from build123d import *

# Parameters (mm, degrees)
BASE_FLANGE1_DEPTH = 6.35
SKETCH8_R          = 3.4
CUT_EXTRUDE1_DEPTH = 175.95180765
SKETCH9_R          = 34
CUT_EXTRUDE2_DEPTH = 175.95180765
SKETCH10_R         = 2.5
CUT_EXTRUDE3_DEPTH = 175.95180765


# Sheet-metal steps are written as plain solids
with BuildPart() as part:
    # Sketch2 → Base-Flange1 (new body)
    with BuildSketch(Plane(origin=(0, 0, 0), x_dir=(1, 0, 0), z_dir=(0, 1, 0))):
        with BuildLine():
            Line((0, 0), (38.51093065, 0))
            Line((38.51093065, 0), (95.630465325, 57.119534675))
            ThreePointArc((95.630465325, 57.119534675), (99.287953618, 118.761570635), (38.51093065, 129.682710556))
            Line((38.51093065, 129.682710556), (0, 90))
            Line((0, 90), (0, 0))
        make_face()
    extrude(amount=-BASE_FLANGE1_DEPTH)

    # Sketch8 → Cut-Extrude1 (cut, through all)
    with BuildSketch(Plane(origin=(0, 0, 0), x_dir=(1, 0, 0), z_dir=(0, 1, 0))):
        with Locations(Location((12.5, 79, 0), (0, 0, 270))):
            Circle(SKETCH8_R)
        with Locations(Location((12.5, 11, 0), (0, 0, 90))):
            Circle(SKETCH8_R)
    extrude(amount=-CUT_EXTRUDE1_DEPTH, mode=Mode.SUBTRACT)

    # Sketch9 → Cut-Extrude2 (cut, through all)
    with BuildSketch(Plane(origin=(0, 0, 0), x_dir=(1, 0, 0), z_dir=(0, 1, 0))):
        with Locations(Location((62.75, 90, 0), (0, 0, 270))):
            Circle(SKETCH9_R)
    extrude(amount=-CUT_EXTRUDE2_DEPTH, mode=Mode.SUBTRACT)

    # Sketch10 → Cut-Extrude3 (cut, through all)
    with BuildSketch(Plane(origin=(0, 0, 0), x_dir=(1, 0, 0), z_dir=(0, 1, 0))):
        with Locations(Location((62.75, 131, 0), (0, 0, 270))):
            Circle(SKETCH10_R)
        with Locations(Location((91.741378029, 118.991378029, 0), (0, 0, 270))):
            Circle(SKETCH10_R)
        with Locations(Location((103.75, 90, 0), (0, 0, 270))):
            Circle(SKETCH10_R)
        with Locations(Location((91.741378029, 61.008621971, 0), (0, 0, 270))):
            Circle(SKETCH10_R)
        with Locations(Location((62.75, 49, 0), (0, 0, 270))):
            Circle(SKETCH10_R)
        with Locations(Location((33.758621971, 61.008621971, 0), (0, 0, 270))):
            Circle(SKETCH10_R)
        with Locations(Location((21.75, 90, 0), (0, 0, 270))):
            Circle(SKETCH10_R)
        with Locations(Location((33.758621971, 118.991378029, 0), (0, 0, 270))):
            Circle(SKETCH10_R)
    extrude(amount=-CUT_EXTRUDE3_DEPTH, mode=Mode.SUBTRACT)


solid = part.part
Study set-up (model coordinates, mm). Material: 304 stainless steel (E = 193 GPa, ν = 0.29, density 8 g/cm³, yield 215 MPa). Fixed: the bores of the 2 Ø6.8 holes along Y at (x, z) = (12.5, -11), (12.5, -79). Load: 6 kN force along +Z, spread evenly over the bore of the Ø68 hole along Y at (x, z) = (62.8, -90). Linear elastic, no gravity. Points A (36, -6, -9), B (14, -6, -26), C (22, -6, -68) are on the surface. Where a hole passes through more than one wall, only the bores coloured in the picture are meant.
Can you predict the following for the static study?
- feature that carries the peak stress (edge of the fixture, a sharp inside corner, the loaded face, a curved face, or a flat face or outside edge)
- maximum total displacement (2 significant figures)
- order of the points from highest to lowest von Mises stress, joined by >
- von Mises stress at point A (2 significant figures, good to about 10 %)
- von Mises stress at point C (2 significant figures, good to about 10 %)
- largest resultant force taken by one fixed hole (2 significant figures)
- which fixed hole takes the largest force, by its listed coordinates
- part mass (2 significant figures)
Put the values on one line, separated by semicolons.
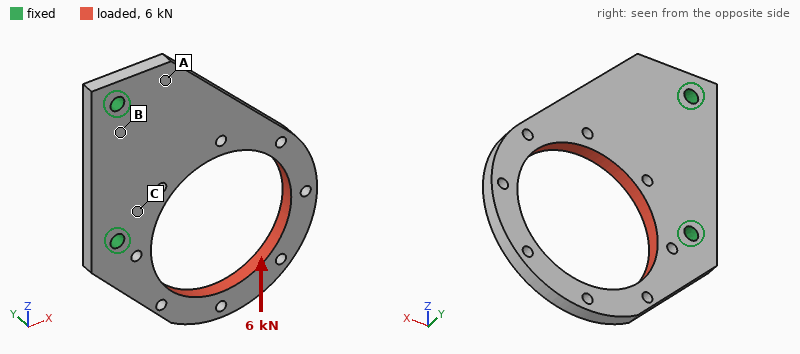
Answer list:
a curved face; 0.12 mm; C > A > B; 26 MPa; 46 MPa; 5.6 kN; (12.5, -79); 350 g
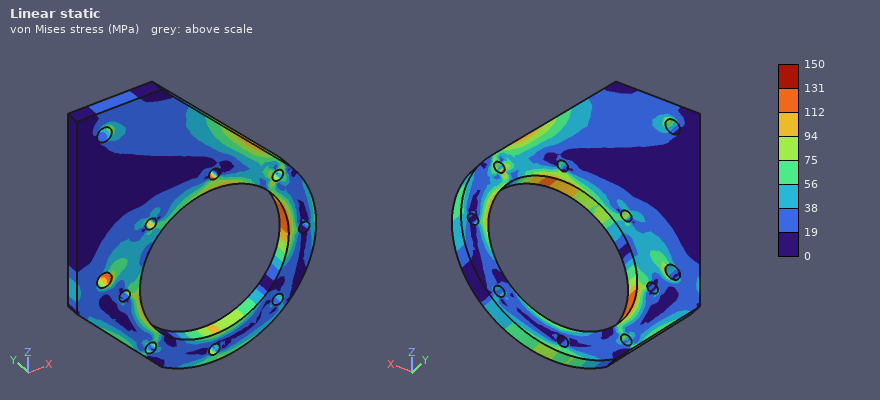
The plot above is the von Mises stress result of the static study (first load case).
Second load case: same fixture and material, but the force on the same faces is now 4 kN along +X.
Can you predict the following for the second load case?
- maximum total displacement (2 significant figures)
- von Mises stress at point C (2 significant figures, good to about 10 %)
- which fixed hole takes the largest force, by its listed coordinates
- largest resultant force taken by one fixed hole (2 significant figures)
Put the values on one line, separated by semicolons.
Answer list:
82 µm; 28 MPa; (12.5, -79); 4.4 kN
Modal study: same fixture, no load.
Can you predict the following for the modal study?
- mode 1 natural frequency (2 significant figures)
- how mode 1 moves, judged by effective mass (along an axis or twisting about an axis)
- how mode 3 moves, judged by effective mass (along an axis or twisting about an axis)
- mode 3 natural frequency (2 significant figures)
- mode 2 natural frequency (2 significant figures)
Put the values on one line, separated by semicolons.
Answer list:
520 Hz; along Y; along Y; 2100 Hz; 1100 Hz
